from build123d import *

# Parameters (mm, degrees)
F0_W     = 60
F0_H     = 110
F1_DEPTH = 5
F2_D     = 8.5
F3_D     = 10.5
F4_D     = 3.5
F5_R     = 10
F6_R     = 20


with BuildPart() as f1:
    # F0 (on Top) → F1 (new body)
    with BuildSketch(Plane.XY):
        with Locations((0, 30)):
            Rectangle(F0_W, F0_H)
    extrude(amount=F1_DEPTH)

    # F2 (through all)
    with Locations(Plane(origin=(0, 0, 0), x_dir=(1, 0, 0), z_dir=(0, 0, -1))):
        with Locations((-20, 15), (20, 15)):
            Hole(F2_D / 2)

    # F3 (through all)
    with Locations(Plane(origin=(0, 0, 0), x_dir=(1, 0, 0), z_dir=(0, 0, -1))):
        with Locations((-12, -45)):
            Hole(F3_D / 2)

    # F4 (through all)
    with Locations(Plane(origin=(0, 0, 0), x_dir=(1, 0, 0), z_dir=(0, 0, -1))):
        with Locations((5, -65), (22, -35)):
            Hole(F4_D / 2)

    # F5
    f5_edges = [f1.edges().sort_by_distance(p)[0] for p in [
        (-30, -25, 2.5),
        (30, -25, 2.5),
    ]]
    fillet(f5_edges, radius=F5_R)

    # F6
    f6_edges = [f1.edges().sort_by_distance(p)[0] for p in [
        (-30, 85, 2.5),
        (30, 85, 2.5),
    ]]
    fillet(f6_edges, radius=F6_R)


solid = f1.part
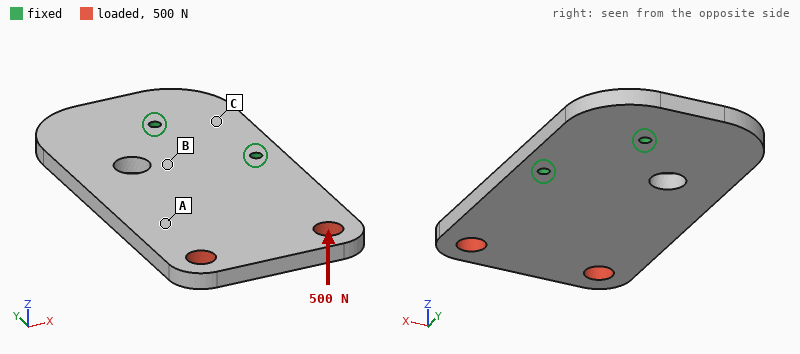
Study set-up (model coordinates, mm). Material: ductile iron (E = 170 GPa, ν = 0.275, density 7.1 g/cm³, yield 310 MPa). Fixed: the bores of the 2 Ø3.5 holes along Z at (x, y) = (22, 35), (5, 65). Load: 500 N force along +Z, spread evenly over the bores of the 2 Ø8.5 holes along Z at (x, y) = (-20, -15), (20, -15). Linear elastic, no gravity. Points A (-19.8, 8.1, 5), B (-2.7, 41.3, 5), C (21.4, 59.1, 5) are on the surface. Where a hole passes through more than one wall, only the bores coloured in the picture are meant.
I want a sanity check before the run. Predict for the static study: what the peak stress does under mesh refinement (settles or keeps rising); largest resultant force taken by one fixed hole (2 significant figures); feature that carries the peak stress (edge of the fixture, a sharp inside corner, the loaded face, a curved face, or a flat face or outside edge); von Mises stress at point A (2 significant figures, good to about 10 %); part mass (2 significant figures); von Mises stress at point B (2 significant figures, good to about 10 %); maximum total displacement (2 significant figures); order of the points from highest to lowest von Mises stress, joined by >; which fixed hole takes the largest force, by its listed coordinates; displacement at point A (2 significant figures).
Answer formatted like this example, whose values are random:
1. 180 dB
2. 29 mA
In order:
1. keeps rising
2. 800 N
3. edge of the fixture
4. 40 MPa
5. 220 g
6. 77 MPa
7. 0.50 mm
8. B > A > C
9. (22, 35)
10. 0.23 mm
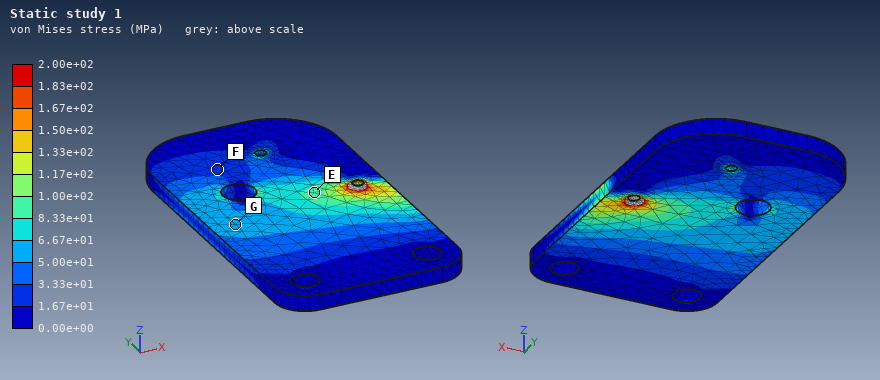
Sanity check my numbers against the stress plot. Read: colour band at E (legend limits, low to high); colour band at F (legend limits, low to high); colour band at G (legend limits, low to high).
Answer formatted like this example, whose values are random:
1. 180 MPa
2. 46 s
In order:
1. 8.33e+01 to 1.00e+02 MPa
2. 1.67e+01 to 3.33e+01 MPa
3. 5.00e+01 to 6.67e+01 MPa
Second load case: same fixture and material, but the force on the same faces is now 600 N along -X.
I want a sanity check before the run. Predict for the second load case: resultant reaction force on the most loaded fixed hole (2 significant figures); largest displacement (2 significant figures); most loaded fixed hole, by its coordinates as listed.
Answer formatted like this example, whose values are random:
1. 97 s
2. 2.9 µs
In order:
1. 1.3 kN
2. 11 µm
3. (22, 35)
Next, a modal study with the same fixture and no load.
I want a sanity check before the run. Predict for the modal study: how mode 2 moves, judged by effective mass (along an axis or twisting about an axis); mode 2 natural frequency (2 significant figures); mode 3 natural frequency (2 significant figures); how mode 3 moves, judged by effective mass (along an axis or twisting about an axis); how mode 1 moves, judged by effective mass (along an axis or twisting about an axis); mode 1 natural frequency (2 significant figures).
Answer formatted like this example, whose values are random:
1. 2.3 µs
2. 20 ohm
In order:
1. twisting about Y
2. 1800 Hz
3. 3300 Hz
4. along Z
5. along Z
6. 780 Hz
